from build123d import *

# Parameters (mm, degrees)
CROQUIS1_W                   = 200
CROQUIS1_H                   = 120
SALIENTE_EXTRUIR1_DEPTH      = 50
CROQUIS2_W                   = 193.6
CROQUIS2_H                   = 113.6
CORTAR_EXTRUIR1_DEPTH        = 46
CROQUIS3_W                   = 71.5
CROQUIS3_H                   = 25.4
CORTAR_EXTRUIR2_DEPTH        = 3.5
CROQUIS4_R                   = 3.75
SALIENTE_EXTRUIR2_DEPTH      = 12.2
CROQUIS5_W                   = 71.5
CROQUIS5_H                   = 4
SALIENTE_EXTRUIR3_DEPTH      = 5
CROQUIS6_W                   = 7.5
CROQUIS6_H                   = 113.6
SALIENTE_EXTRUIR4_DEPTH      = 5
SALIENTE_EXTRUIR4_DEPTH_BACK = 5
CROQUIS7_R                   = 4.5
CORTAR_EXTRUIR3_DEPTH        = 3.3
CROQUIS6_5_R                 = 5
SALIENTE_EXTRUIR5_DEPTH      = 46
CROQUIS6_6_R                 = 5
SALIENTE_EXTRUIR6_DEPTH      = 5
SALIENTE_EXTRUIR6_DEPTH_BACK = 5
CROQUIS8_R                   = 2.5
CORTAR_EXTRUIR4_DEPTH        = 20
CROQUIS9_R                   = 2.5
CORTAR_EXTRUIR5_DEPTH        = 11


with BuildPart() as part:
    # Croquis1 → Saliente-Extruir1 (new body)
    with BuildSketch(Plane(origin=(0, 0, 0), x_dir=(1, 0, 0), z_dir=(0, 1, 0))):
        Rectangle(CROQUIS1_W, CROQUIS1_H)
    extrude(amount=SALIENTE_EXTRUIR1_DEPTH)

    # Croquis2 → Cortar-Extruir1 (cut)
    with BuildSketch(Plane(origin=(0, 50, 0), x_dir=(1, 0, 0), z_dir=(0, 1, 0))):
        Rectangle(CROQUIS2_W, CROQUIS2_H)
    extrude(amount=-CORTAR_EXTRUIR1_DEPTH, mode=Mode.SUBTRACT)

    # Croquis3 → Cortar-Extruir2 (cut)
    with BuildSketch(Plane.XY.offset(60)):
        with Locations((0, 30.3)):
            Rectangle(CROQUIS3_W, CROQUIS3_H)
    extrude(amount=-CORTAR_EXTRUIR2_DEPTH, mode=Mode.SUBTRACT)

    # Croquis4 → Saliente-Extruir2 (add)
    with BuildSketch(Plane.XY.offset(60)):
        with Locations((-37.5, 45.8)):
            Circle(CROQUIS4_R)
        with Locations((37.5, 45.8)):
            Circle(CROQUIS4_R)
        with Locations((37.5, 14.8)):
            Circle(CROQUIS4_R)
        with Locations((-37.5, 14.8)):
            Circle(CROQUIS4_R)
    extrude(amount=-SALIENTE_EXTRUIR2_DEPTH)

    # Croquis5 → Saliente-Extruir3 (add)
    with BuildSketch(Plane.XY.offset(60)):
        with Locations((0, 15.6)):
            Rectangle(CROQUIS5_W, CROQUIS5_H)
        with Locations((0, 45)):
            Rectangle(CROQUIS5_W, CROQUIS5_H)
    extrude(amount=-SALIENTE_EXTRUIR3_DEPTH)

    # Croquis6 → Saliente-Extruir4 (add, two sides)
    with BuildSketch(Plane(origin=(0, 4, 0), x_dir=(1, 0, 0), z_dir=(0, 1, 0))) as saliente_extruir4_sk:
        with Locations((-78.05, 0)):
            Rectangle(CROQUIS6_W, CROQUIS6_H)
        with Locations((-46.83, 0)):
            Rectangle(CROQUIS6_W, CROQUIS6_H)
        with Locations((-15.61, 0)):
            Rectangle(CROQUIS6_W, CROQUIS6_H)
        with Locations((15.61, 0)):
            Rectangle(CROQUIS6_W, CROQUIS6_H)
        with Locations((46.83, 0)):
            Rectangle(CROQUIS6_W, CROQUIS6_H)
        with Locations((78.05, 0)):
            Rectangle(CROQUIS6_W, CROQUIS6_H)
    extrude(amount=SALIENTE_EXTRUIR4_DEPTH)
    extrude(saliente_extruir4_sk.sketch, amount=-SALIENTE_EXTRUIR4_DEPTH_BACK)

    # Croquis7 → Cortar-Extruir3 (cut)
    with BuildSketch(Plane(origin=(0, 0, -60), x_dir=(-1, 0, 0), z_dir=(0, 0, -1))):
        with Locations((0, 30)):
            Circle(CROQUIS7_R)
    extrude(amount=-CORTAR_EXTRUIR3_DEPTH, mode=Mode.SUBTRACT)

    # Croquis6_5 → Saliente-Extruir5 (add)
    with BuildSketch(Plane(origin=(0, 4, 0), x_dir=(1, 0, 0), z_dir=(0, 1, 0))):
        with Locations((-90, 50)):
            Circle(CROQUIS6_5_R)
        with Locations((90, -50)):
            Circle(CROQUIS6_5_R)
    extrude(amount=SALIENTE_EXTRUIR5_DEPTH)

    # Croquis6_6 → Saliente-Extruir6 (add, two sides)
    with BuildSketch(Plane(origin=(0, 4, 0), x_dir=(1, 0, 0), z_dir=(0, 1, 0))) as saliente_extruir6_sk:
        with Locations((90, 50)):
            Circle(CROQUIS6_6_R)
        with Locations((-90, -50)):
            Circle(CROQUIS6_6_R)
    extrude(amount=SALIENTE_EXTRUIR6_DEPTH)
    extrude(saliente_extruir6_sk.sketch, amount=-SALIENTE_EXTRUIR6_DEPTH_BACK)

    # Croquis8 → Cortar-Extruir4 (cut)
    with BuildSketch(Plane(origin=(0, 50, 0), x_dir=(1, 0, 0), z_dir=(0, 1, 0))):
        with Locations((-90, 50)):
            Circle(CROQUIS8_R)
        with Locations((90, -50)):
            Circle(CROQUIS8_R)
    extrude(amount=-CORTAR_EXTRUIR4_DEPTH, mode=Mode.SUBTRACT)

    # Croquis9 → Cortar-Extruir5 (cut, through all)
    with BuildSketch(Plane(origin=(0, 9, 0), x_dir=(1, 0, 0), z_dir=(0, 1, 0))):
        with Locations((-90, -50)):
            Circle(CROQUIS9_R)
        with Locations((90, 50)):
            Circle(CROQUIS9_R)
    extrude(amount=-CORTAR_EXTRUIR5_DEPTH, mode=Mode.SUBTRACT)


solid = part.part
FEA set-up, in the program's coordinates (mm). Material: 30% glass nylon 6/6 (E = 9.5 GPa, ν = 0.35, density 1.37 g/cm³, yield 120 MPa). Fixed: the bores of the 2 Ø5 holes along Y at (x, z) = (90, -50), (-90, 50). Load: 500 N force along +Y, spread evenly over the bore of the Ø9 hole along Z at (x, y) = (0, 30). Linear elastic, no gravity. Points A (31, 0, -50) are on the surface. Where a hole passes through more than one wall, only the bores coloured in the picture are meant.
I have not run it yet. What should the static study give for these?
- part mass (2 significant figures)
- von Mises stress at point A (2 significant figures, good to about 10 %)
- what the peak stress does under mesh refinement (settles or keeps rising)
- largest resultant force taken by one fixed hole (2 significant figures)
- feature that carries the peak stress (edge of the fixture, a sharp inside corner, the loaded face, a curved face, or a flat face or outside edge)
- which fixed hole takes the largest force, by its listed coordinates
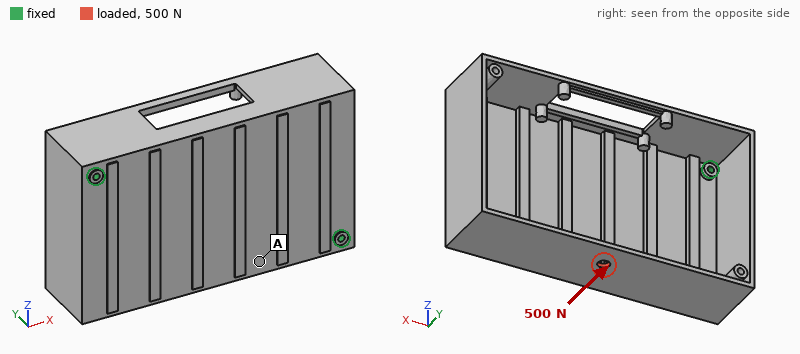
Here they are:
300 g
4.5 MPa
keeps rising
330 N
edge of the fixture
(90, -50)
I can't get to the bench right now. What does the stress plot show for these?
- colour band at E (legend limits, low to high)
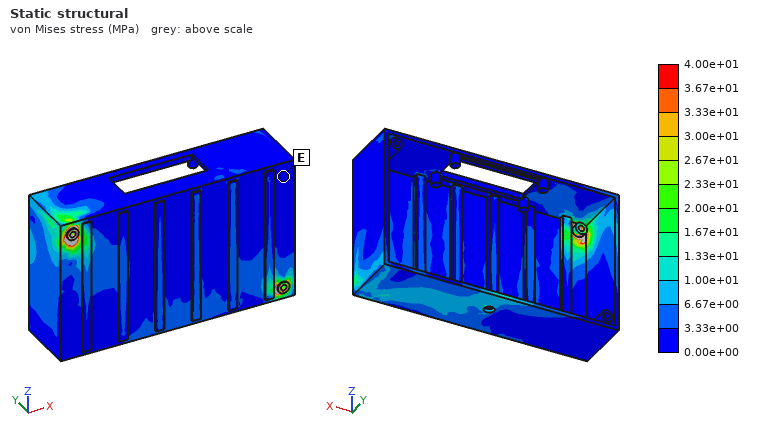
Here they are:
0.00e+00 to 3.33e+00 MPa
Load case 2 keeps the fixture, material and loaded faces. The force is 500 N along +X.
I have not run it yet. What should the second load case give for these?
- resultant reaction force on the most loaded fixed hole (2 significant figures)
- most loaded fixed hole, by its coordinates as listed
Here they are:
390 N
(90, -50)
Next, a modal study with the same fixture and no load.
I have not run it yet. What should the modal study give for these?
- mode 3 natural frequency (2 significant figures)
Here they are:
600 Hz
